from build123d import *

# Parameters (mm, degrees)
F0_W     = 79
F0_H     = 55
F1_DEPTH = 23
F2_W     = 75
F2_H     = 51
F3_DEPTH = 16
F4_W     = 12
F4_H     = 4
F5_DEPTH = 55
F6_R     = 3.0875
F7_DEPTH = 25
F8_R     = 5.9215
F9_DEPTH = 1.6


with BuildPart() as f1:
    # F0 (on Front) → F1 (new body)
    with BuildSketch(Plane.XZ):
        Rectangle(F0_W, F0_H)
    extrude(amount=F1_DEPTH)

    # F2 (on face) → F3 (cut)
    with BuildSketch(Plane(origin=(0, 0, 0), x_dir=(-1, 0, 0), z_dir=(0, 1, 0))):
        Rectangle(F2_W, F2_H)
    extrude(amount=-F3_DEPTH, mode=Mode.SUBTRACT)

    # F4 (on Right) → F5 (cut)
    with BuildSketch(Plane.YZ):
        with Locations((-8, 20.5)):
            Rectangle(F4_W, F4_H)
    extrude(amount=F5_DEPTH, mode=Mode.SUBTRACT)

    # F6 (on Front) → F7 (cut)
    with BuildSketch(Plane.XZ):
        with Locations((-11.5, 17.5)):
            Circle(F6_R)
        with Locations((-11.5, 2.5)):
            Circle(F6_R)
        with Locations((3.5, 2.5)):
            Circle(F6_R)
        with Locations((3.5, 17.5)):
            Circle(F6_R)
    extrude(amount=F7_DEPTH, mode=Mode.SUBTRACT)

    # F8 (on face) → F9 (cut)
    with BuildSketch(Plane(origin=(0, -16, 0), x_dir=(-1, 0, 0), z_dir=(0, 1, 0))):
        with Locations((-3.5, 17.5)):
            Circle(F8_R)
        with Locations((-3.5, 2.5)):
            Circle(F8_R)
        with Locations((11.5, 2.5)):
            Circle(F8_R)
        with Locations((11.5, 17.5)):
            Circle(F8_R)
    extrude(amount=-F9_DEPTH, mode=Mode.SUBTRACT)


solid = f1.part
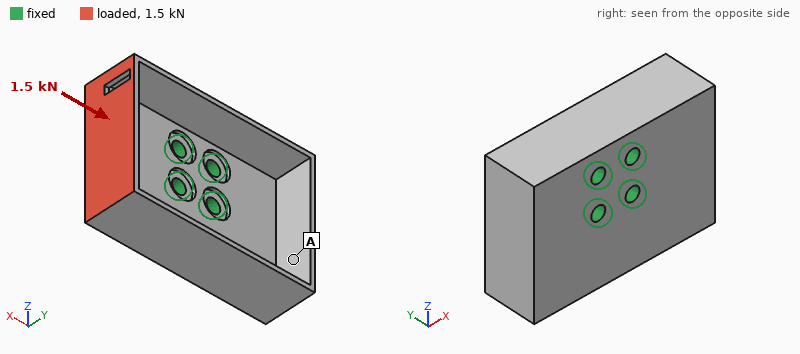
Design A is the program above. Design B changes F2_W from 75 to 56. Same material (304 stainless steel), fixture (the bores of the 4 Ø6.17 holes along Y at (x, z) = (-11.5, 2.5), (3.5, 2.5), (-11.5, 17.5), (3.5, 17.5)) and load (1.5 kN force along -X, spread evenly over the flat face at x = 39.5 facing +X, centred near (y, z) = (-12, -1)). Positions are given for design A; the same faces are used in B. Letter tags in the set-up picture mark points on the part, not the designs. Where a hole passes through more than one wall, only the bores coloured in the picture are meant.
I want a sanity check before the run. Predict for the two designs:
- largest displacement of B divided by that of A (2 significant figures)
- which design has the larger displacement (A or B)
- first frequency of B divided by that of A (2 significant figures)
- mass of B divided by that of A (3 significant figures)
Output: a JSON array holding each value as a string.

["0.20", "A", "0.86", "1.40"]
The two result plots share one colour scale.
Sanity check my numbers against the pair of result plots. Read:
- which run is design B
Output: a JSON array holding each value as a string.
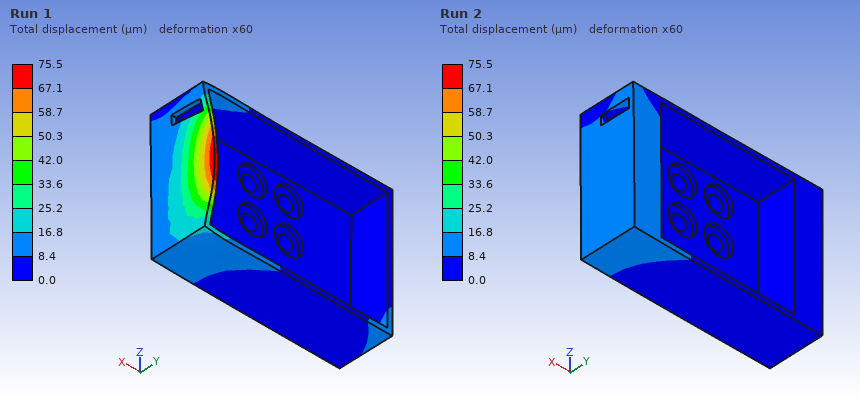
["Run 2"]
